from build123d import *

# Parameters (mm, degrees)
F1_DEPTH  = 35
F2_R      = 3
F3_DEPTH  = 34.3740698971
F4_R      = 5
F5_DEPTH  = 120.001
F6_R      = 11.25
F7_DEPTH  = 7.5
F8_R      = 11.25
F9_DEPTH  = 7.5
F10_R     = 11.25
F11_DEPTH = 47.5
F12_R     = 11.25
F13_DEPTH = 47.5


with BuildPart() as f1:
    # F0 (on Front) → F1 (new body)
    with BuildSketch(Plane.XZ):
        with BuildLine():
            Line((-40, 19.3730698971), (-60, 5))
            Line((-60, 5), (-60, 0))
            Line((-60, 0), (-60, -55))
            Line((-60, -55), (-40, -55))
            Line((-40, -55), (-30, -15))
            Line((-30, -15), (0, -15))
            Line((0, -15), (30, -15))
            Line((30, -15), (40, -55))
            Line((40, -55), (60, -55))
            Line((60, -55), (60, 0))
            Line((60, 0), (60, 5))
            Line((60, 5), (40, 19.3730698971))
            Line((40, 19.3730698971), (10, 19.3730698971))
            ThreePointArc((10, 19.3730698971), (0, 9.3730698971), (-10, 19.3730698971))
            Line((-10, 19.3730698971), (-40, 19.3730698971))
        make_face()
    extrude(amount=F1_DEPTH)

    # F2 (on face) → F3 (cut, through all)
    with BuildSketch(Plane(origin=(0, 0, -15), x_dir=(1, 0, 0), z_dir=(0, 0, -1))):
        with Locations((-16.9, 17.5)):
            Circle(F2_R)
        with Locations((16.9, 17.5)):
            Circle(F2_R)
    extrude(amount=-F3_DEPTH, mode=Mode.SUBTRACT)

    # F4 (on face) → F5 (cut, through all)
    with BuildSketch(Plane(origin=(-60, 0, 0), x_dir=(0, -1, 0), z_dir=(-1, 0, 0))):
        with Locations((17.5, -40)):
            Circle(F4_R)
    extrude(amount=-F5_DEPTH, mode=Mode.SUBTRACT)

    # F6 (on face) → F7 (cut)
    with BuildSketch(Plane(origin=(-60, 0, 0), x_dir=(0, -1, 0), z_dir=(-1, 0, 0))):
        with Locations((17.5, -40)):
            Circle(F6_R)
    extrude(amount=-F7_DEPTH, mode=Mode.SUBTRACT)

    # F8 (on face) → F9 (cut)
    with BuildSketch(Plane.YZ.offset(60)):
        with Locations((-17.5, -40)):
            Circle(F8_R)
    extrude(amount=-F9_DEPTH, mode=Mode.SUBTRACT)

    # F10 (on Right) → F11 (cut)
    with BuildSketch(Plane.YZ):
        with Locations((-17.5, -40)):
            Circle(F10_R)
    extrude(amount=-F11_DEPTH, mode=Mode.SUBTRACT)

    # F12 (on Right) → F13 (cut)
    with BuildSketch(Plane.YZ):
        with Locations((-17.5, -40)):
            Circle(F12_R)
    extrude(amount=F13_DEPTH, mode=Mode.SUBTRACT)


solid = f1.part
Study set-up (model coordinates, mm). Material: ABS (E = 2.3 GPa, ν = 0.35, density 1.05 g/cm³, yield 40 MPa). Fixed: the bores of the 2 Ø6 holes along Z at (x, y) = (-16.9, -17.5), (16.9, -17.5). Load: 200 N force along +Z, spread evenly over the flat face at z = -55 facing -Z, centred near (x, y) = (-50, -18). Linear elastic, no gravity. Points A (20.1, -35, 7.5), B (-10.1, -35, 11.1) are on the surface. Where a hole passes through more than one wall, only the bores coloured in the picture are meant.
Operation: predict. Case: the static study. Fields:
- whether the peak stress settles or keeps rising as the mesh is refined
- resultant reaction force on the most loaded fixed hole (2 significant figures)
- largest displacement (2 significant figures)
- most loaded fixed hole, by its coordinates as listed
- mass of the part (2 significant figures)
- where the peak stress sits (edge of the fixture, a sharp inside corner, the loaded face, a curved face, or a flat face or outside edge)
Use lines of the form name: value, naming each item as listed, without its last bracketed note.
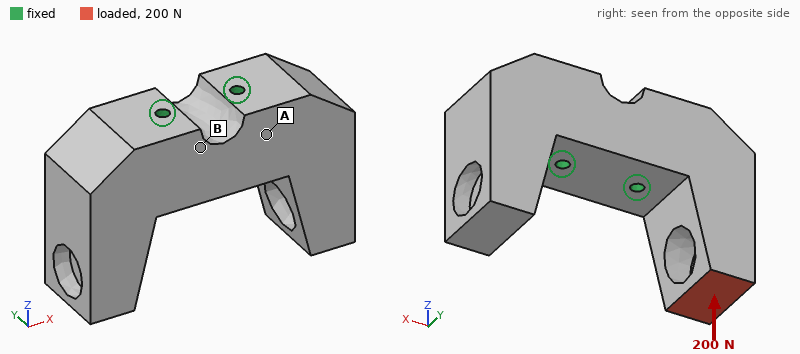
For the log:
whether the peak stress settles or keeps rising as the mesh is refined: keeps rising
resultant reaction force on the most loaded fixed hole: 230 N
largest displacement: 66 µm
most loaded fixed hole, by its coordinates as listed: (-16.9, -17.5)
mass of the part: 190 g
where the peak stress sits: edge of the fixture
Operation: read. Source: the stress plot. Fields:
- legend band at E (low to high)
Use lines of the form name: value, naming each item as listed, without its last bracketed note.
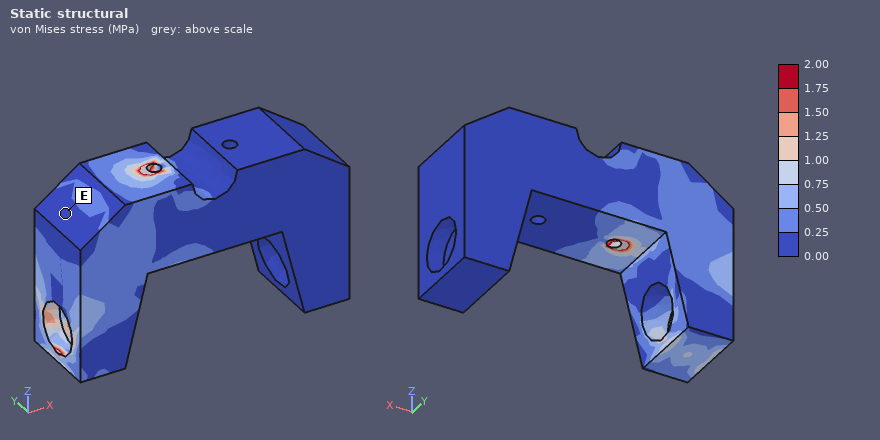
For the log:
legend band at E: 0.00 to 0.25 MPa
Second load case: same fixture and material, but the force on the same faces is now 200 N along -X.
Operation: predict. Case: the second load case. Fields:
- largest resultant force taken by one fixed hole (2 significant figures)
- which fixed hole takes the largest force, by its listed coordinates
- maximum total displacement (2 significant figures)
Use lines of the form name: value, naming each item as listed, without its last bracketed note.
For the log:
largest resultant force taken by one fixed hole: 150 N
which fixed hole takes the largest force, by its listed coordinates: (-16.9, -17.5)
maximum total displacement: 0.20 mm
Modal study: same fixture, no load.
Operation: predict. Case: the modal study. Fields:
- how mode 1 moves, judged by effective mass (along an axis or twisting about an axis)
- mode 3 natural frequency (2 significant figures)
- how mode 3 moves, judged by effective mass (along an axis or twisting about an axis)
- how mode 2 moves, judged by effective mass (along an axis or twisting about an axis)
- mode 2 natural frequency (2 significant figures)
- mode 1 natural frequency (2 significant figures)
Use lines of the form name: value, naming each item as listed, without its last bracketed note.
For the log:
how mode 1 moves, judged by effective mass: twisting about Z
mode 3 natural frequency: 1600 Hz
how mode 3 moves, judged by effective mass: along X
how mode 2 moves, judged by effective mass: along Y
mode 2 natural frequency: 1400 Hz
mode 1 natural frequency: 1300 Hz
